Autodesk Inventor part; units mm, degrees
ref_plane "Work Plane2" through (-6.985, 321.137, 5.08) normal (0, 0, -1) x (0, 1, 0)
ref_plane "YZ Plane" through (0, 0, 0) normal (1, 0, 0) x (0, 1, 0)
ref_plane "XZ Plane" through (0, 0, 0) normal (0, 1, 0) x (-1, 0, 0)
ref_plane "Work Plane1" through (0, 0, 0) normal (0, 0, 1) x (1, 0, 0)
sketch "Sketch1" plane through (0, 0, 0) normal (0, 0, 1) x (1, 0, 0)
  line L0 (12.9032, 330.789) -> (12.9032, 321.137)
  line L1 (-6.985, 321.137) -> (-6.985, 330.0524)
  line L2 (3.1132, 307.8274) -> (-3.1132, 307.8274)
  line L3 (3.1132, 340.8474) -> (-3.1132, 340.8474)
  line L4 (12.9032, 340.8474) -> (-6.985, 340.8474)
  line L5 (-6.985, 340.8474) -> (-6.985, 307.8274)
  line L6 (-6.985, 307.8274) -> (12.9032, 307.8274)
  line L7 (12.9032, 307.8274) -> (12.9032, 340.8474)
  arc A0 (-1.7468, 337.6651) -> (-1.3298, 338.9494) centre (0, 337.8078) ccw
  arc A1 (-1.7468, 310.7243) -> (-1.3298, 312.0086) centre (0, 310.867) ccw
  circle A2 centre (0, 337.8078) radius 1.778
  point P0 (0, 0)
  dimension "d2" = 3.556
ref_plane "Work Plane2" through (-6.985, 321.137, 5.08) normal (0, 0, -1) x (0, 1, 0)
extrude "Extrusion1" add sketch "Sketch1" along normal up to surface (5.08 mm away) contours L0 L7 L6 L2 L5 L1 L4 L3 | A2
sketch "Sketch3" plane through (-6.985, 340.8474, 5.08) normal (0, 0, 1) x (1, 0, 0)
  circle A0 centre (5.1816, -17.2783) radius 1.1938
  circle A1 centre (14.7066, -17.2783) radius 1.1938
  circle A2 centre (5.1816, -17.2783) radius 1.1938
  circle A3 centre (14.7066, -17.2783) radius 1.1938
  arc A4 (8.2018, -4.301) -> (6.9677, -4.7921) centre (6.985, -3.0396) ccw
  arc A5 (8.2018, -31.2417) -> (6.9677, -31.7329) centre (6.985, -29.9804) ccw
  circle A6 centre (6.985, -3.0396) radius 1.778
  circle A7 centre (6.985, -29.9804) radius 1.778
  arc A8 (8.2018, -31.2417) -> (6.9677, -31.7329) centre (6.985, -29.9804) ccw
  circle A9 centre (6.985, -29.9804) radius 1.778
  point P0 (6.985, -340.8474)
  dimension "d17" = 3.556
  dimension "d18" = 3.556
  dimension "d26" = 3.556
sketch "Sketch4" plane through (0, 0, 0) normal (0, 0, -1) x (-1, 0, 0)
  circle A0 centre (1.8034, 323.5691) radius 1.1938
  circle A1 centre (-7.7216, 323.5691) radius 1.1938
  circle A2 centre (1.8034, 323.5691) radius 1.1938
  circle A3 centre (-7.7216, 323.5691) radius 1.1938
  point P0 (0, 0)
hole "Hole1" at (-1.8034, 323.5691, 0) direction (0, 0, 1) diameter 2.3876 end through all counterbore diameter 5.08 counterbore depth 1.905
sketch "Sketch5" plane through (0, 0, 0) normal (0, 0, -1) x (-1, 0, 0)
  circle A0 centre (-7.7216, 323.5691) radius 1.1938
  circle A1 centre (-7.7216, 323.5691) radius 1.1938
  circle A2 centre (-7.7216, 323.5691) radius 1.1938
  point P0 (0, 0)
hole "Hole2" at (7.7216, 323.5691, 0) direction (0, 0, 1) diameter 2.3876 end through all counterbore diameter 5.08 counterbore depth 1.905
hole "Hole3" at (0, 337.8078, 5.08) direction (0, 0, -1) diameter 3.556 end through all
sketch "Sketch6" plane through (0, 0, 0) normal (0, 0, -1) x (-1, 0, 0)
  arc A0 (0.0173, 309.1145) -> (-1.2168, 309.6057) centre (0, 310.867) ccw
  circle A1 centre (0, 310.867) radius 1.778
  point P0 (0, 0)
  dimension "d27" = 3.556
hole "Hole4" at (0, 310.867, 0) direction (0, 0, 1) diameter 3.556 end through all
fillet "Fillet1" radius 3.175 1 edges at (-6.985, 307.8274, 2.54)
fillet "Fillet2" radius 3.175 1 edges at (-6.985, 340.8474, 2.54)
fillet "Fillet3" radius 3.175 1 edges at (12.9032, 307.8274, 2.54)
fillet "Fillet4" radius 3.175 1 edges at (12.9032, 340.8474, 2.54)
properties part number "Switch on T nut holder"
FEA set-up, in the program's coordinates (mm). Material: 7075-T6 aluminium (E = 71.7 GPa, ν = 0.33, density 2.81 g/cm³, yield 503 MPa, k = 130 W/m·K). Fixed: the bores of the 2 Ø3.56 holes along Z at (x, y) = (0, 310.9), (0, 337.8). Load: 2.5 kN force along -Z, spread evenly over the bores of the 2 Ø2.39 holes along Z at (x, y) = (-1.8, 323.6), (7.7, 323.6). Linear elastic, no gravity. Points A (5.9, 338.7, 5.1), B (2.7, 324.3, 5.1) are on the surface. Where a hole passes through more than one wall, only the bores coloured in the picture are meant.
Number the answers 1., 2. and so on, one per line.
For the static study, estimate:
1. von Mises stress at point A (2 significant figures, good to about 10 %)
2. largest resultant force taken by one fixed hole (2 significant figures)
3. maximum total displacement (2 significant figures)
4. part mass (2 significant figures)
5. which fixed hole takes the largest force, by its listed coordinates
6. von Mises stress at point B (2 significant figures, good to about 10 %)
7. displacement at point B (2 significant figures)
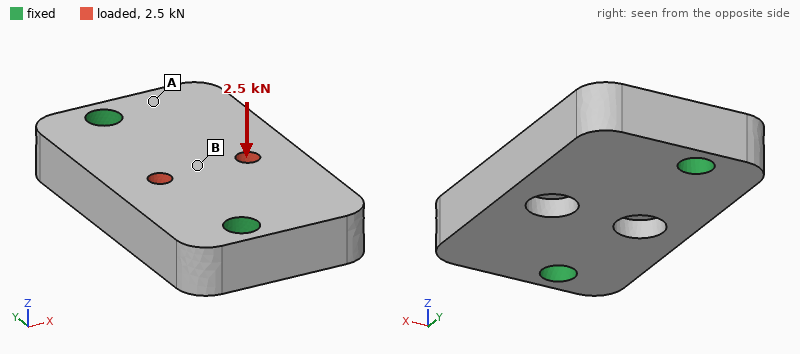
1. 46 MPa
2. 1.4 kN
3. 56 µm
4. 8.7 g
5. (0, 310.9)
6. 120 MPa
7. 34 µm
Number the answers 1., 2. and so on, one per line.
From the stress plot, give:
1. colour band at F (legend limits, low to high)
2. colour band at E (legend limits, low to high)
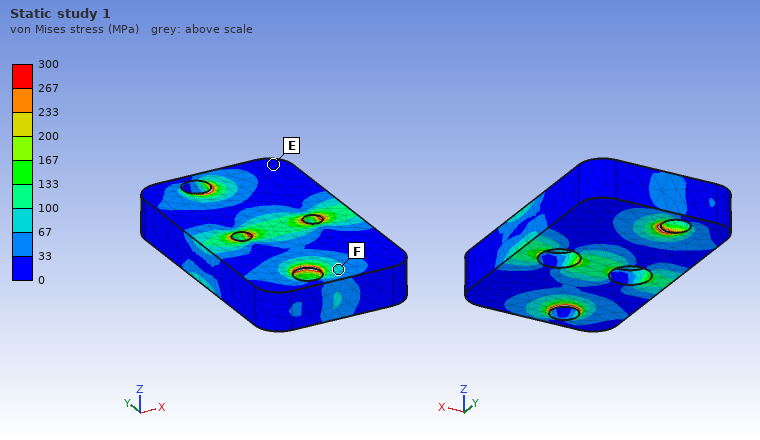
1. 67 to 100 MPa
2. 0 to 33 MPa
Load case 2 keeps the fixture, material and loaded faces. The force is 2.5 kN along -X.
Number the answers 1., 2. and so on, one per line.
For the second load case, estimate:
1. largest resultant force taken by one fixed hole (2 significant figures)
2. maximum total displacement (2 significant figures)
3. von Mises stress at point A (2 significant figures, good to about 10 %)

1. 1.4 kN
2. 16 µm
3. 17 MPa
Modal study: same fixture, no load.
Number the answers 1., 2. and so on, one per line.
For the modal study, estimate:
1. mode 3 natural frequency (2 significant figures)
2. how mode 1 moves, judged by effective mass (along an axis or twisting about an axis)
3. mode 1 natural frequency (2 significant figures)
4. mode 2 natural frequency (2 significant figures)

1. 31 kHz
2. along Z
3. 18 kHz
4. 30 kHz
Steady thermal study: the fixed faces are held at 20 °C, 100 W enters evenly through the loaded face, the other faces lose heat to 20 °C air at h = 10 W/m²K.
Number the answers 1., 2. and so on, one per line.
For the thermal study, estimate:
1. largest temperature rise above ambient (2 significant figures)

1. 77 K
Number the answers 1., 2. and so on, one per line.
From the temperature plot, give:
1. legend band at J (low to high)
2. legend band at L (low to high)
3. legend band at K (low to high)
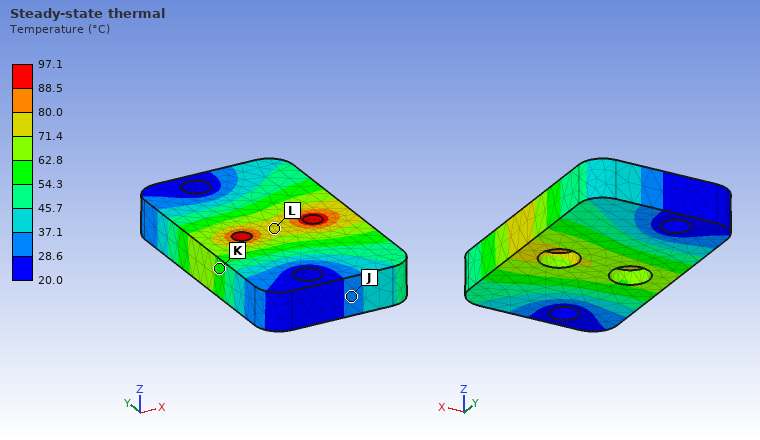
1. 28.6 to 37.1 °C
2. 71.4 to 80.0 °C
3. 54.3 to 62.8 °C
